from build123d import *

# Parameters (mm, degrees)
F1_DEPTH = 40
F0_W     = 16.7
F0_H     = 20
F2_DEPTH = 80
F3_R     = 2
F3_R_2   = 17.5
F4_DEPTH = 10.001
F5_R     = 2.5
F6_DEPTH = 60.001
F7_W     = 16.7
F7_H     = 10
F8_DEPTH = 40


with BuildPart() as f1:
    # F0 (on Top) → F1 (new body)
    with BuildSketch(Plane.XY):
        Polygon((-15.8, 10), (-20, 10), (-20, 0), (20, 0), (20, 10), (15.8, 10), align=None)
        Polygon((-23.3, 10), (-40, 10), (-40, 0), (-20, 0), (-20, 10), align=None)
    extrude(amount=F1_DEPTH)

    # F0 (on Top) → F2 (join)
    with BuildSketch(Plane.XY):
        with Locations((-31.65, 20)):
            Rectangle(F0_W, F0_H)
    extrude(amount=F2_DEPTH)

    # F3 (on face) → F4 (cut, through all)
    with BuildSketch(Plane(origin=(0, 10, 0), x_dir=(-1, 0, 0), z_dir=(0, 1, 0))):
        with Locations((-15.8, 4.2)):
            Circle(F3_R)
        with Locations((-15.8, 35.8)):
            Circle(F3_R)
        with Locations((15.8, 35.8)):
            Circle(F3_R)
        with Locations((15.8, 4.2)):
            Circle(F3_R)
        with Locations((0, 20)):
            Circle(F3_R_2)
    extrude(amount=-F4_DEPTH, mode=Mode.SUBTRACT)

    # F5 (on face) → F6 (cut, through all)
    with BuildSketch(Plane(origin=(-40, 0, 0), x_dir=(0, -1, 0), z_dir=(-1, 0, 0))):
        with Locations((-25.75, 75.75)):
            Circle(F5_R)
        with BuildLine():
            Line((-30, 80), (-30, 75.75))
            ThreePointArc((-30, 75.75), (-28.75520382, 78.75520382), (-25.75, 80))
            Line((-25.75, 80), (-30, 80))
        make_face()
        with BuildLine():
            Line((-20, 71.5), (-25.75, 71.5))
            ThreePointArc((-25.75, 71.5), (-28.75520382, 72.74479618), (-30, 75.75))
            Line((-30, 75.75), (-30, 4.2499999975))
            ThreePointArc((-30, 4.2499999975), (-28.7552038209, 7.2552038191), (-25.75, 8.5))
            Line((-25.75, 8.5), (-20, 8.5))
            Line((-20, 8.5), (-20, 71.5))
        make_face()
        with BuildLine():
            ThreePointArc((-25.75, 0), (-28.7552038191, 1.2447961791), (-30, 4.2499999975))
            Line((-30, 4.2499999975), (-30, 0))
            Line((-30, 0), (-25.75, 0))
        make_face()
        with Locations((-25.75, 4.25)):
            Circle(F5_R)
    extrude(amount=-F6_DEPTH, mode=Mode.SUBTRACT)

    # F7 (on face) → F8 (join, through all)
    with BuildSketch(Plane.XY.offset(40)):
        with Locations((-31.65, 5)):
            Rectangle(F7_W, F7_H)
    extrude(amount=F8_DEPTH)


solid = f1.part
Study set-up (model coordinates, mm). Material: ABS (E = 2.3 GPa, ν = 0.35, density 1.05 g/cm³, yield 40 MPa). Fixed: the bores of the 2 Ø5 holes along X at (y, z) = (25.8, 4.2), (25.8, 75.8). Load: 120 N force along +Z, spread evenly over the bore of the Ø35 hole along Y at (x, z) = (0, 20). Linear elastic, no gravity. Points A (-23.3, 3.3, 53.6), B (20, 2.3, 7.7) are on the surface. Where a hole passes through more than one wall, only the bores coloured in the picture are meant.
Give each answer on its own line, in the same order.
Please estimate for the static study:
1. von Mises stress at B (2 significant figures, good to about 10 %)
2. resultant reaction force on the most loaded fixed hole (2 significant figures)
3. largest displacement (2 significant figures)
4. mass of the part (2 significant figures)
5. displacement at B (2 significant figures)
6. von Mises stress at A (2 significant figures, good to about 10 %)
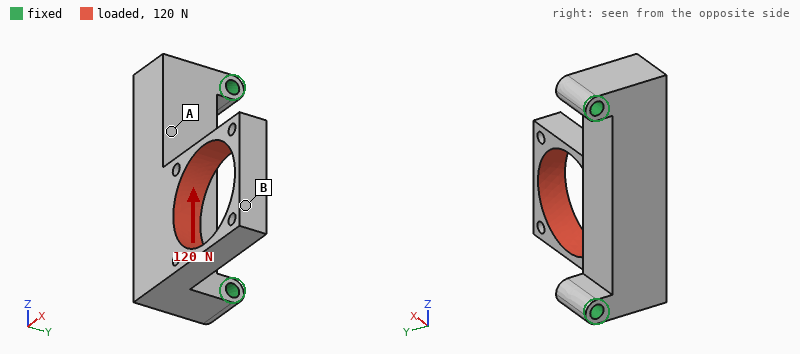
3.6 MPa
85 N
0.56 mm
38 g
0.54 mm
0.99 MPa
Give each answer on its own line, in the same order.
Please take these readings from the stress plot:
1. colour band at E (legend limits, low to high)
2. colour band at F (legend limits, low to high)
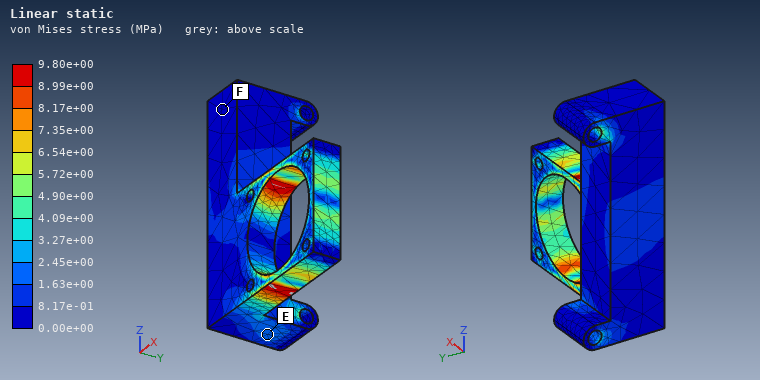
1.63e+00 to 2.45e+00 MPa
0.00e+00 to 8.17e-01 MPa
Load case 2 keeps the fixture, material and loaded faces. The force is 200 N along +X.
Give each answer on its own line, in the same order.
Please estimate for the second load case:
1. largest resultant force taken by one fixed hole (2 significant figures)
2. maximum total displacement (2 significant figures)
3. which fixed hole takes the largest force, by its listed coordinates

160 N
0.30 mm
(25.8, 4.2)
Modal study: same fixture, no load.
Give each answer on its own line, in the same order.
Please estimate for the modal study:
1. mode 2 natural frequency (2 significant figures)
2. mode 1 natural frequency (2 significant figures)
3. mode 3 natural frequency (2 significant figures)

1000 Hz
750 Hz
1400 Hz
